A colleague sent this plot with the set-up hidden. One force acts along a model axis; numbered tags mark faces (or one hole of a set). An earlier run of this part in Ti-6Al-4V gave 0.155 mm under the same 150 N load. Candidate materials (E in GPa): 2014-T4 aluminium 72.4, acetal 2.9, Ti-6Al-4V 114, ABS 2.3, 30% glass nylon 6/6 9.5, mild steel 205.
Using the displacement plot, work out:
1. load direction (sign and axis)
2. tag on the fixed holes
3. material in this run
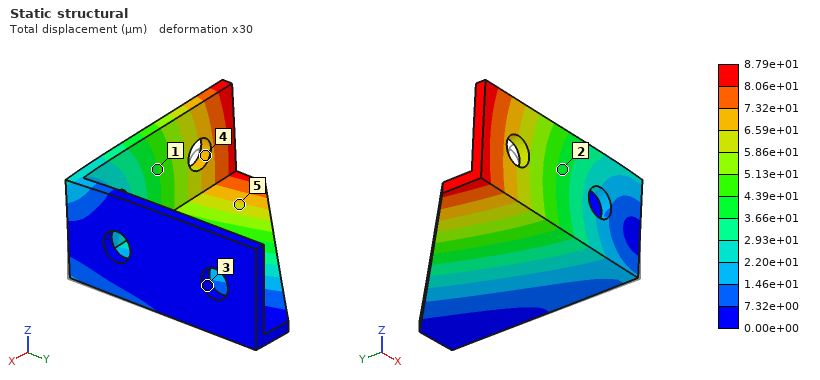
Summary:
+Z
3
mild steel
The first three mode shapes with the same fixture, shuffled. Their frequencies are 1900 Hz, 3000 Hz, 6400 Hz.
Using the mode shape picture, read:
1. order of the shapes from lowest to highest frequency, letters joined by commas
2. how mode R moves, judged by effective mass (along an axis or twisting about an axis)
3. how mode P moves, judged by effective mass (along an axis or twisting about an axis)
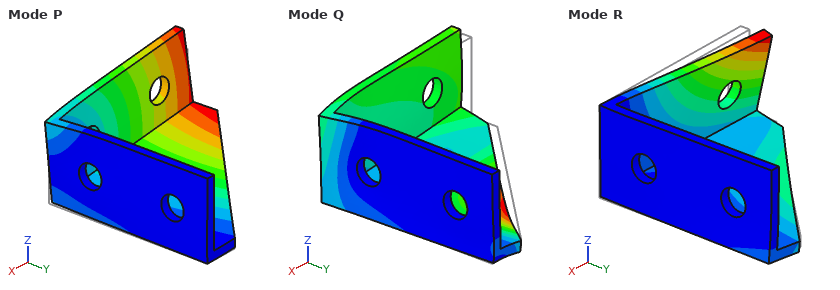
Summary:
P, R, Q
along Y
along Z
